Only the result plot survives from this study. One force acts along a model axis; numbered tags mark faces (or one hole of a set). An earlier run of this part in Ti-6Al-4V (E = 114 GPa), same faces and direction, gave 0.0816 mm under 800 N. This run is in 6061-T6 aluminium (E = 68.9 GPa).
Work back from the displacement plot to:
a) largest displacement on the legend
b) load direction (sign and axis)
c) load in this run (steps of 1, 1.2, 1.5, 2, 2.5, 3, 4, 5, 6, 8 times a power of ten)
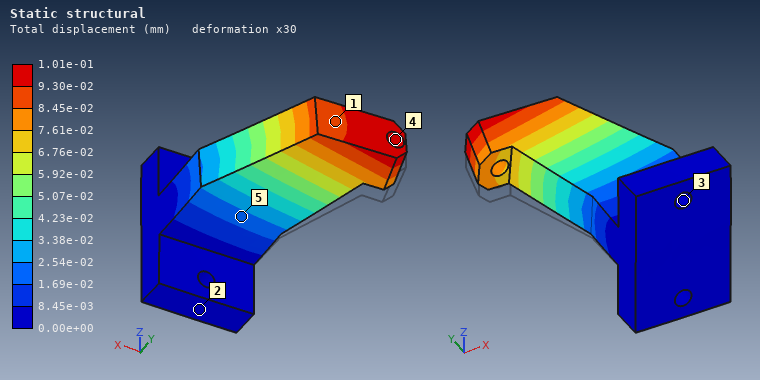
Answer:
1.01e-01 mm
+Z
600 N
